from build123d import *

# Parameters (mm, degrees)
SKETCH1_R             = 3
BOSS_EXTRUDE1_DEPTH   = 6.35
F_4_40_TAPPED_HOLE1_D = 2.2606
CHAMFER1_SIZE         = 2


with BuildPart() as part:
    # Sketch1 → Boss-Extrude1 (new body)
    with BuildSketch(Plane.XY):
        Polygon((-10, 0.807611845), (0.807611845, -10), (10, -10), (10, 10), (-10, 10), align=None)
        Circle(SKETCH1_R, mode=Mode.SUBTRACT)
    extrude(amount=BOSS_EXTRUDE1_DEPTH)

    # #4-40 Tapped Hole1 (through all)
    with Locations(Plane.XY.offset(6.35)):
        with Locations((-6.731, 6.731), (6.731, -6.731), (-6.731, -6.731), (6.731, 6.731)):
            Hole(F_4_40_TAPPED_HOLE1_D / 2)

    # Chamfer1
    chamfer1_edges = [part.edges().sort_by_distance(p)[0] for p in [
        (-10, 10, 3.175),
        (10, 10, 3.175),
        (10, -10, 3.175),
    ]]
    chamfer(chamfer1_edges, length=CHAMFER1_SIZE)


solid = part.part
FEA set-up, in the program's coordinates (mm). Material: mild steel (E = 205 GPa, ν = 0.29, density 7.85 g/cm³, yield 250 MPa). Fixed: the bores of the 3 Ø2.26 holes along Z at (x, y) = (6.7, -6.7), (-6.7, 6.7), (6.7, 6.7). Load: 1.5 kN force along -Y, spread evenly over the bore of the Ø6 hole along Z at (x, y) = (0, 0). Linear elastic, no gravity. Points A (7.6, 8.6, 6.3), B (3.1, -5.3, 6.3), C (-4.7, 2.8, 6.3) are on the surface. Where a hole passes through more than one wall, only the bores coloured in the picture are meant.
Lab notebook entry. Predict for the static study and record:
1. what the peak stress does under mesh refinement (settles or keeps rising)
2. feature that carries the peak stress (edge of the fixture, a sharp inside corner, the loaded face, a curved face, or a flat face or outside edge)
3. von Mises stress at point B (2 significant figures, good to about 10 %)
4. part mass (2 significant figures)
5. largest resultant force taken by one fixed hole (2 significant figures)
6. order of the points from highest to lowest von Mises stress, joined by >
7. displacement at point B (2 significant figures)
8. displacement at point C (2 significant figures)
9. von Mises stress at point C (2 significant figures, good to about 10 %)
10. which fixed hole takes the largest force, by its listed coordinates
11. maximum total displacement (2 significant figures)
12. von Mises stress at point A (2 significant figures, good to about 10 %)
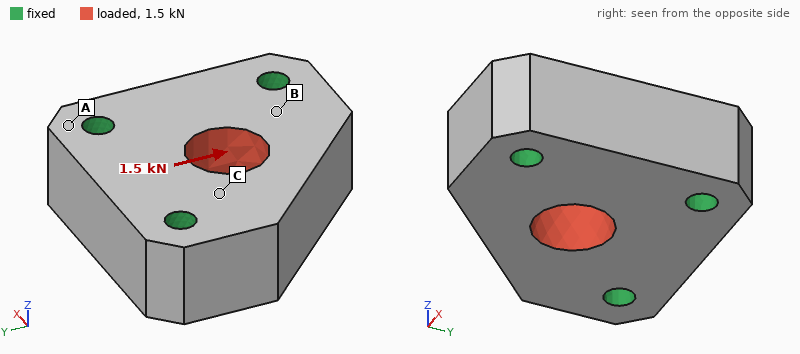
keeps rising
edge of the fixture
11 MPa
15 g
650 N
C > B > A
0.42 µm
0.41 µm
17 MPa
(-6.7, 6.7)
1.1 µm
5.4 MPa
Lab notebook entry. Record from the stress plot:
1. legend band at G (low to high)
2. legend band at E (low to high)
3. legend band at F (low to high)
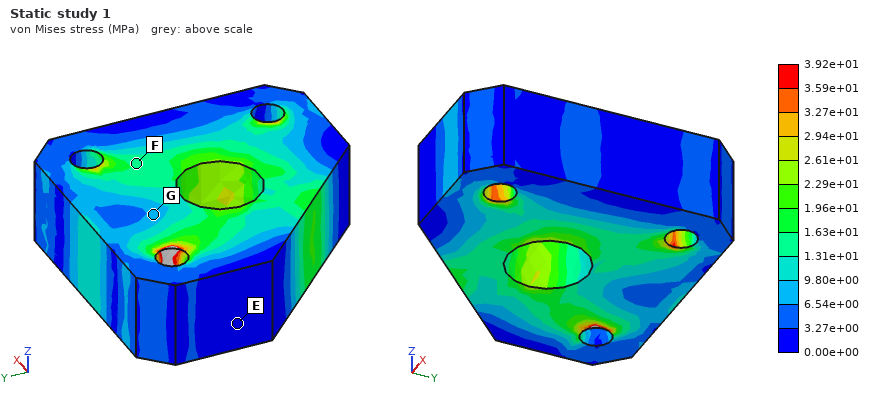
6.54e+00 to 9.80e+00 MPa
0.00e+00 to 3.27e+00 MPa
1.31e+01 to 1.63e+01 MPa
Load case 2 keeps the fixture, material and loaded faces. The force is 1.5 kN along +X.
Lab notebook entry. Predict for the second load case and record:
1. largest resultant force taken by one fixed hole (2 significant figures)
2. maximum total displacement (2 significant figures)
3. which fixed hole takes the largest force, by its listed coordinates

650 N
1.1 µm
(6.7, -6.7)
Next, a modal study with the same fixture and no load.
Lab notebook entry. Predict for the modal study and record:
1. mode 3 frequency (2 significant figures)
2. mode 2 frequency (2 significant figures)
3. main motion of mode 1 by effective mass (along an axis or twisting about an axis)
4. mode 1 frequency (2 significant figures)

89 kHz
84 kHz
along Z
52 kHz
